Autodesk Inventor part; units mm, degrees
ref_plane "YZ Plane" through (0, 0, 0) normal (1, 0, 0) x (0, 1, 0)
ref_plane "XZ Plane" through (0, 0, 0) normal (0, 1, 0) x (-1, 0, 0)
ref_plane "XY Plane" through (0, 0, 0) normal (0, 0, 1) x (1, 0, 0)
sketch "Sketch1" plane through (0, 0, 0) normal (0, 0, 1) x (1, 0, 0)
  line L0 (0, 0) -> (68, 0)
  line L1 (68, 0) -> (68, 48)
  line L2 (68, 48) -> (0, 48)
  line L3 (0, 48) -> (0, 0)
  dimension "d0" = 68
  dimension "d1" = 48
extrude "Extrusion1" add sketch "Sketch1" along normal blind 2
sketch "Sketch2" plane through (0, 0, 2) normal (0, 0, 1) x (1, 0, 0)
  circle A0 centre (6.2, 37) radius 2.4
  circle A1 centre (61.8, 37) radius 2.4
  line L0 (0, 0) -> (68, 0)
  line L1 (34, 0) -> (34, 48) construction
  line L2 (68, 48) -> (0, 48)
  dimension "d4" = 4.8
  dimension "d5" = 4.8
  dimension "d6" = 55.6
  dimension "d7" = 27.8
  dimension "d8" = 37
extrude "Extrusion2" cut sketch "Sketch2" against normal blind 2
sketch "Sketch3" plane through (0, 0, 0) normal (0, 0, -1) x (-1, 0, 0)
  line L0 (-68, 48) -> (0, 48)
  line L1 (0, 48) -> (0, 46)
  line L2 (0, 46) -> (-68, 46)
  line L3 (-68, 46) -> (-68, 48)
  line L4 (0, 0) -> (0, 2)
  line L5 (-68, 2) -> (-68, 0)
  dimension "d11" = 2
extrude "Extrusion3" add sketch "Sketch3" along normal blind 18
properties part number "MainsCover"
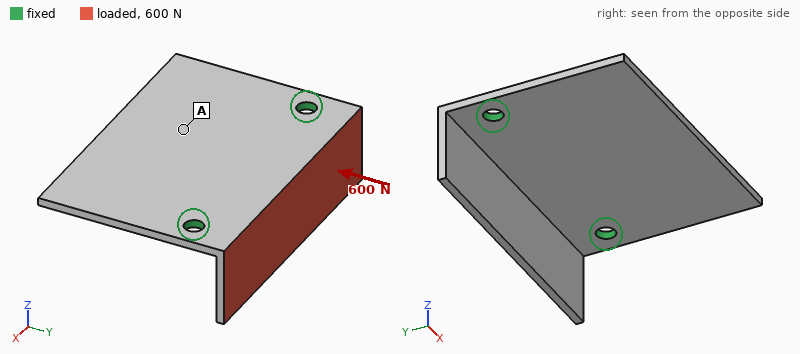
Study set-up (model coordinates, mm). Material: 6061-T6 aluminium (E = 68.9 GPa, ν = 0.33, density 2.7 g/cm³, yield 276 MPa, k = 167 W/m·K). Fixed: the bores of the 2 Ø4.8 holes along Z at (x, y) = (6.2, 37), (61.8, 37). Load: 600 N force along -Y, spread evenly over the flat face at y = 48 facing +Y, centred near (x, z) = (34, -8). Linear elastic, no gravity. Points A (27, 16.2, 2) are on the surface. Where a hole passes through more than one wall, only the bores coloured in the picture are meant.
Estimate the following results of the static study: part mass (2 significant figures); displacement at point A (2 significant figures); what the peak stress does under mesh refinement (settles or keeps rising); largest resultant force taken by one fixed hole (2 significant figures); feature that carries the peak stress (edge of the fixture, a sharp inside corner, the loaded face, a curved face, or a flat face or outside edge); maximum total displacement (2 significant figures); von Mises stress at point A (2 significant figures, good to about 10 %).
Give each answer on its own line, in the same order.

24 g
0.14 mm
keeps rising
300 N
edge of the fixture
0.50 mm
18 MPa
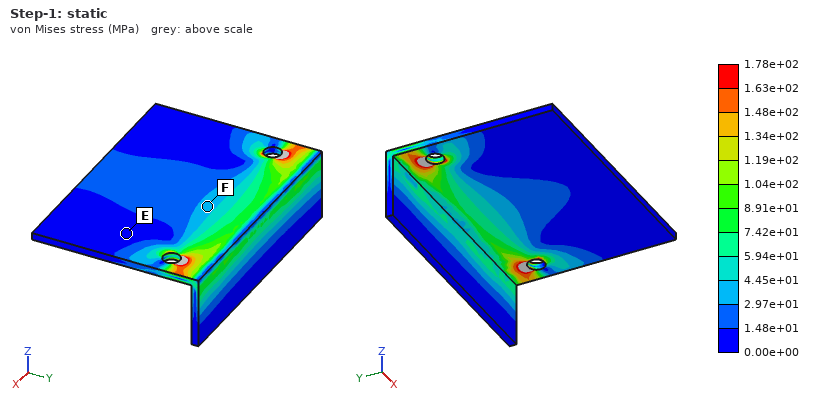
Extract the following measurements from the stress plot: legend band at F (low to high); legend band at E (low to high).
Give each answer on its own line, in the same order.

2.97e+01 to 4.45e+01 MPa
0.00e+00 to 1.48e+01 MPa
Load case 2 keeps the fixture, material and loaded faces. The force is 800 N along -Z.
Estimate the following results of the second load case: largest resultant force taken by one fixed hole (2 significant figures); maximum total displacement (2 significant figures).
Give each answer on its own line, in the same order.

430 N
0.39 mm
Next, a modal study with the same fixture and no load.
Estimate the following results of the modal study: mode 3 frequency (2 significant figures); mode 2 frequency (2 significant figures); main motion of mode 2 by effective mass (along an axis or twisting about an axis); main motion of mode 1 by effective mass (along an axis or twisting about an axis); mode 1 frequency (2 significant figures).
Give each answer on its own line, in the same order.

2500 Hz
2000 Hz
twisting about Y
along Z
1000 Hz
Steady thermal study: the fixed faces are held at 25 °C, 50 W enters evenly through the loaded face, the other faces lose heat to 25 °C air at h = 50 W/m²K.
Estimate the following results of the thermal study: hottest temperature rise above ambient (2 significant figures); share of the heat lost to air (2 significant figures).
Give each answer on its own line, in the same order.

52 K
16 %
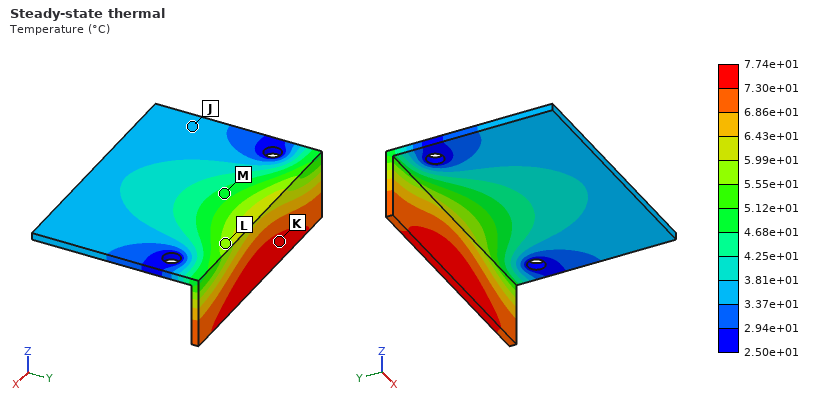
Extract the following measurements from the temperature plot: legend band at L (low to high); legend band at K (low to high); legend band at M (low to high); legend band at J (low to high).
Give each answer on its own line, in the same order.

5.55e+01 to 5.99e+01 °C
7.30e+01 to 7.74e+01 °C
4.68e+01 to 5.12e+01 °C
3.37e+01 to 3.81e+01 °C
